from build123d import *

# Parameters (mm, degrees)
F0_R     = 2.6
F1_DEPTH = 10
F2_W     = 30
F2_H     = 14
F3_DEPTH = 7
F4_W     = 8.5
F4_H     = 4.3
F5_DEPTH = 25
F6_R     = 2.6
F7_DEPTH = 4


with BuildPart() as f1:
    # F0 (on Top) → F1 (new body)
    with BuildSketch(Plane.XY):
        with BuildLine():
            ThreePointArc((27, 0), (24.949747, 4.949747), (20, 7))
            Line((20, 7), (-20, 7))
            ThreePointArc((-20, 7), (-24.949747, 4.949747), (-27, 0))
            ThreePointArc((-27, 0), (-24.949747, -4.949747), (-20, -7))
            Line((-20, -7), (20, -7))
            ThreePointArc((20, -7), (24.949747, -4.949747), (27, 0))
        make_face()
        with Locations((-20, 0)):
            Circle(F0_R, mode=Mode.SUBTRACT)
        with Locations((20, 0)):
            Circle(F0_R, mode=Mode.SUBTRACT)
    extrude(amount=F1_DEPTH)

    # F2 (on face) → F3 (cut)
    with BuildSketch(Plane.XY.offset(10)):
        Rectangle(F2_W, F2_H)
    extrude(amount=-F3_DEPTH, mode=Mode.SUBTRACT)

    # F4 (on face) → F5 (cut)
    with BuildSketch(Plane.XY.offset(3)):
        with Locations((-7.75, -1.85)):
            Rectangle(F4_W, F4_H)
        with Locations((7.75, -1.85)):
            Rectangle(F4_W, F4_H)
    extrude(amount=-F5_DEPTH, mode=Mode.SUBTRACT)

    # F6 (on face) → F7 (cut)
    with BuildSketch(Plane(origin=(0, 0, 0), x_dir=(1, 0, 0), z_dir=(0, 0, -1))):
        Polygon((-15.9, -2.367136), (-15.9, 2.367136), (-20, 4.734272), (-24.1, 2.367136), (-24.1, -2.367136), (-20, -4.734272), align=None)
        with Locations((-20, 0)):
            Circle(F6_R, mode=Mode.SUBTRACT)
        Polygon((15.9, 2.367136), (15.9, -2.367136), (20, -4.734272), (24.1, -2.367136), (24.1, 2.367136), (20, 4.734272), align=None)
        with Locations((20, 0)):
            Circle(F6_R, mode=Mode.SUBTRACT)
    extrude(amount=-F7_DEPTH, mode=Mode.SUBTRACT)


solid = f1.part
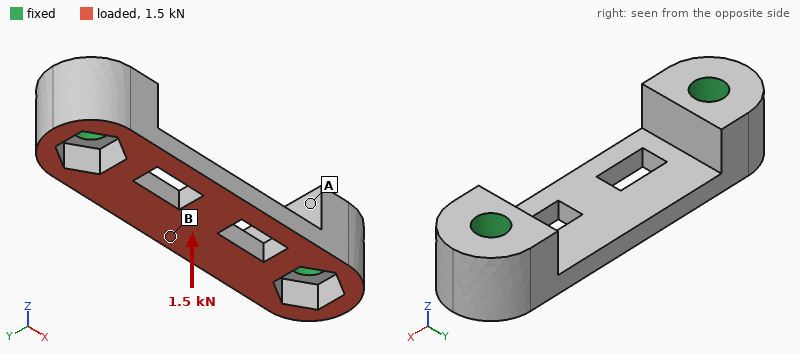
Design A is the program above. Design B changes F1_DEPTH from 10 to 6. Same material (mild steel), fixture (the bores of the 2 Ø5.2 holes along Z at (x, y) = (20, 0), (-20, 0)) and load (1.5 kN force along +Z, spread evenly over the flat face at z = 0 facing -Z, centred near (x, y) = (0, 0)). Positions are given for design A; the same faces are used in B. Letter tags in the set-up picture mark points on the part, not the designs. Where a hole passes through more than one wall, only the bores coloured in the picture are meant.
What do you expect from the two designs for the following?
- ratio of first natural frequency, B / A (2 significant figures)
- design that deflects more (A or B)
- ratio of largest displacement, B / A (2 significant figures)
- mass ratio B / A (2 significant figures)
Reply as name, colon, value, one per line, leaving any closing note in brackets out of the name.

ratio of first natural frequency, B / A: 0.94
design that deflects more: B
ratio of largest displacement, B / A: 1.1
mass ratio B / A: 0.69
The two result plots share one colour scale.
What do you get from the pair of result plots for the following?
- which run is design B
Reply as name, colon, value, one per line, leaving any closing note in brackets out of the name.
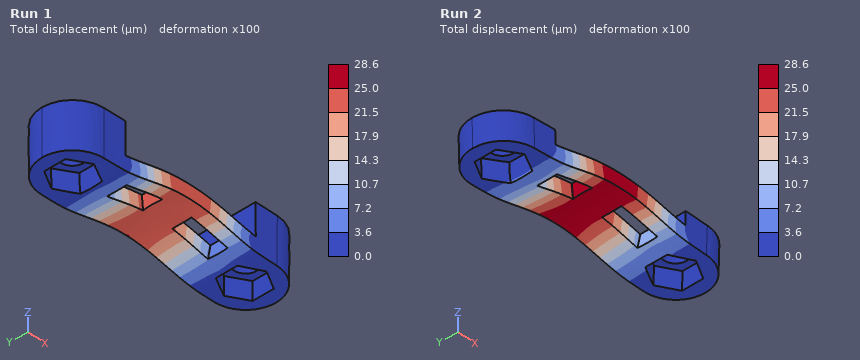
which run is design B: Run 2
